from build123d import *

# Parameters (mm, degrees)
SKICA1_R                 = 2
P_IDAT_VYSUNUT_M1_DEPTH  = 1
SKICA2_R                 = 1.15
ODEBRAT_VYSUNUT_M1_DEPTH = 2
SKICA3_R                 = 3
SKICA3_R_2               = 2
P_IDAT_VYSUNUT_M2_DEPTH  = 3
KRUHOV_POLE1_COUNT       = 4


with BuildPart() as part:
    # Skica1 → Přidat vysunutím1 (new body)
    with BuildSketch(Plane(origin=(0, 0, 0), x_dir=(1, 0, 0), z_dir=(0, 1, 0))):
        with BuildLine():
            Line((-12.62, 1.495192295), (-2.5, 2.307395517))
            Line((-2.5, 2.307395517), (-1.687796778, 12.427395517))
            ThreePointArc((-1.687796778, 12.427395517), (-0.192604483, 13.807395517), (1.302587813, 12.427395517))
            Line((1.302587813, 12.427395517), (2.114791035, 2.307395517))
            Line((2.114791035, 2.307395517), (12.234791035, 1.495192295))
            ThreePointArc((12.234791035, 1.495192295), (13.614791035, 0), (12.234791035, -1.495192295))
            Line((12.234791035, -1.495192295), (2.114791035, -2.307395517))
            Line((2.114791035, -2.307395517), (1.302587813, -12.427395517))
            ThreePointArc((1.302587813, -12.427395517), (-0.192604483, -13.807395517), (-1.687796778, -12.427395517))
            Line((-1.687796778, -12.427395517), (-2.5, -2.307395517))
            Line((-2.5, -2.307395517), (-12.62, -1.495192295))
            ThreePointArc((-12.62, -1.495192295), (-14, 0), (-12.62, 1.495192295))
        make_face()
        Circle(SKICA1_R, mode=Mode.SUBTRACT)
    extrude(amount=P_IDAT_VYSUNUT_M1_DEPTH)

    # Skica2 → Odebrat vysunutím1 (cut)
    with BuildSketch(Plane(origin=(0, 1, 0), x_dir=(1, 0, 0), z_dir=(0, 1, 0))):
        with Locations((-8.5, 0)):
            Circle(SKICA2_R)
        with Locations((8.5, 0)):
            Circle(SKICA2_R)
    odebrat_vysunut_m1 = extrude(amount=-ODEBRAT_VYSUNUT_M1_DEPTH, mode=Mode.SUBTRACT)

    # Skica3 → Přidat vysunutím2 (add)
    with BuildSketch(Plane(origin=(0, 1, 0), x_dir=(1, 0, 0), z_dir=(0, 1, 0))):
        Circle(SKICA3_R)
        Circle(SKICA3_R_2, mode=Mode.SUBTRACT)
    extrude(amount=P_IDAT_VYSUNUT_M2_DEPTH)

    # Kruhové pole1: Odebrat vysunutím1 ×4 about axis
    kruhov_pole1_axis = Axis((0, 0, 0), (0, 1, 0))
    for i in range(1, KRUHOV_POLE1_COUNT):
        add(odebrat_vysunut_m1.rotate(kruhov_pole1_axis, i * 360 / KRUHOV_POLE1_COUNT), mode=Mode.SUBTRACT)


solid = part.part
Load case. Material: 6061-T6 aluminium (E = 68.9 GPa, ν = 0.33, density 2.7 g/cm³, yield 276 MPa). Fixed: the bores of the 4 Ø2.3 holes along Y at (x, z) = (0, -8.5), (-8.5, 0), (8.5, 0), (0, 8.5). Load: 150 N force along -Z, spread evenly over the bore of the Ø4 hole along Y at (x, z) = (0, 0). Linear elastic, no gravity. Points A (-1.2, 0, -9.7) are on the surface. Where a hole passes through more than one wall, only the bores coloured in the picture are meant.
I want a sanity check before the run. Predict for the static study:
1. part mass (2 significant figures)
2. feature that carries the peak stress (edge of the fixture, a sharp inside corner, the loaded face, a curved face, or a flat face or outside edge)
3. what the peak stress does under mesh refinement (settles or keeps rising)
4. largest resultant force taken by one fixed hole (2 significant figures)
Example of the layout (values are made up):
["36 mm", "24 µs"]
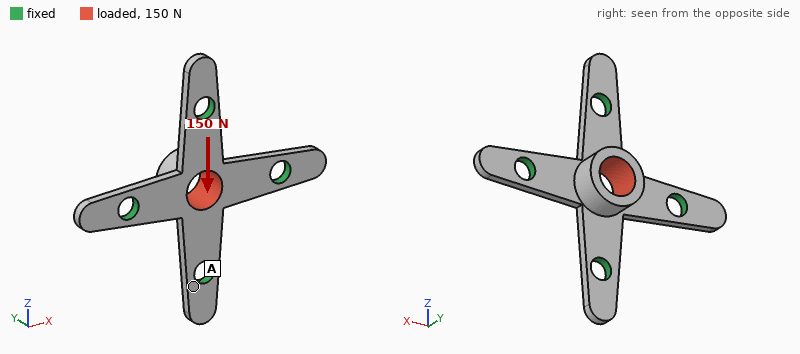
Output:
["0.56 g", "edge of the fixture", "keeps rising", "68 N"]
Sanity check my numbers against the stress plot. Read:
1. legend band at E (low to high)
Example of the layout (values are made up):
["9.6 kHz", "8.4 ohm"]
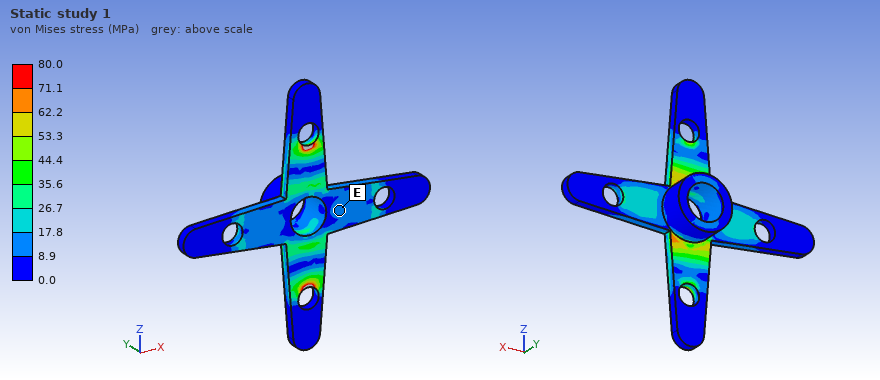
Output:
["8.9 to 17.8 MPa"]
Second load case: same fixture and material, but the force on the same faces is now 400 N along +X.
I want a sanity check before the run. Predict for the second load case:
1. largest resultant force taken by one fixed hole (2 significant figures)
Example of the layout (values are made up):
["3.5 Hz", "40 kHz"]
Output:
["180 N"]
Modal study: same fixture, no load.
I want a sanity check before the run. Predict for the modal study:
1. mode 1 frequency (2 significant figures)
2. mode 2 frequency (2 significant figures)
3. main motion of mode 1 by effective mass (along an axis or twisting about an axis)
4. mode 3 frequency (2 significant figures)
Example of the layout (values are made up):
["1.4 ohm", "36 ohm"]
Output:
["26 kHz", "41 kHz", "along Y", "41 kHz"]
